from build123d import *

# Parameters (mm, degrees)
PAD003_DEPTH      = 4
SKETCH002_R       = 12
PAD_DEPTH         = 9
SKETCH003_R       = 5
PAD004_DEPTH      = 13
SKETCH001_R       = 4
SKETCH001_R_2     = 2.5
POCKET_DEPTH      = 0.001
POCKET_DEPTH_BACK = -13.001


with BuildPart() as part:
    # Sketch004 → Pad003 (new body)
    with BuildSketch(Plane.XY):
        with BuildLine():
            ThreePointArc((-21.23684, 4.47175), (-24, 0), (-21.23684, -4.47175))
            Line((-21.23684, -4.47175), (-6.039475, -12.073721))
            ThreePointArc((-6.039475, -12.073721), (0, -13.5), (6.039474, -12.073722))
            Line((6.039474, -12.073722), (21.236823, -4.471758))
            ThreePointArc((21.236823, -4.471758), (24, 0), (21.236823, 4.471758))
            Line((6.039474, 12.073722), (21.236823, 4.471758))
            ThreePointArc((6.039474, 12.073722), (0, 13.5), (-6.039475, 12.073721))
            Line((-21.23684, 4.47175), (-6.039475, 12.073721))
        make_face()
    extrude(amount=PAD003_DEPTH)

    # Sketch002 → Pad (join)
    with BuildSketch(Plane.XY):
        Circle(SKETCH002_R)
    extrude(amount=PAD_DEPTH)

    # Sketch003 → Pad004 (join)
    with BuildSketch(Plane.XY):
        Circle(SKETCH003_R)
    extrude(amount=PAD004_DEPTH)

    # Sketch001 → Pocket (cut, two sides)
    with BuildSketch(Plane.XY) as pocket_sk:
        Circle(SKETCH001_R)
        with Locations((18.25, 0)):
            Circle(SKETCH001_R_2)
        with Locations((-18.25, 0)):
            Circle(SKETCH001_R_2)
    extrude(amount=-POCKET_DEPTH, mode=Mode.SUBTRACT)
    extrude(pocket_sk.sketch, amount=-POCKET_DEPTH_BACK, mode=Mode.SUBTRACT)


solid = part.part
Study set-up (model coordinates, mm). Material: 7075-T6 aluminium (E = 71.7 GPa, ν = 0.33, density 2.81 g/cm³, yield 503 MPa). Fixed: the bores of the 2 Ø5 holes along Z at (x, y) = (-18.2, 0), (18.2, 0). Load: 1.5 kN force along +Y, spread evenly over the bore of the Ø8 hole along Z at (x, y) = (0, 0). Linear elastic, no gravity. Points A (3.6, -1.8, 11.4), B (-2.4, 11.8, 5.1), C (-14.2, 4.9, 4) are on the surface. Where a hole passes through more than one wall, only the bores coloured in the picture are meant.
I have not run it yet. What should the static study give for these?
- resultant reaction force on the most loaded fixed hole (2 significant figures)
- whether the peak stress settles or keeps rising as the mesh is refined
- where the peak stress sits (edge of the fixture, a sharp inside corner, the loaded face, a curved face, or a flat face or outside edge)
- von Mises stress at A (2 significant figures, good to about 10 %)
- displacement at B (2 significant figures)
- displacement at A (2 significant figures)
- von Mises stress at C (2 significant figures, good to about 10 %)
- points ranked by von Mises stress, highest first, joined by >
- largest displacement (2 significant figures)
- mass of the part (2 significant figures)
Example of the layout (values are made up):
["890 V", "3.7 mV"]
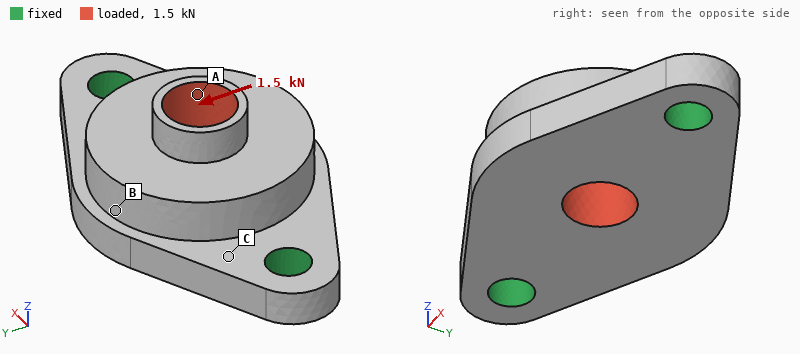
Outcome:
["750 N", "keeps rising", "edge of the fixture", "31 MPa", "31 µm", "31 µm", "58 MPa", "C > A > B", "40 µm", "15 g"]
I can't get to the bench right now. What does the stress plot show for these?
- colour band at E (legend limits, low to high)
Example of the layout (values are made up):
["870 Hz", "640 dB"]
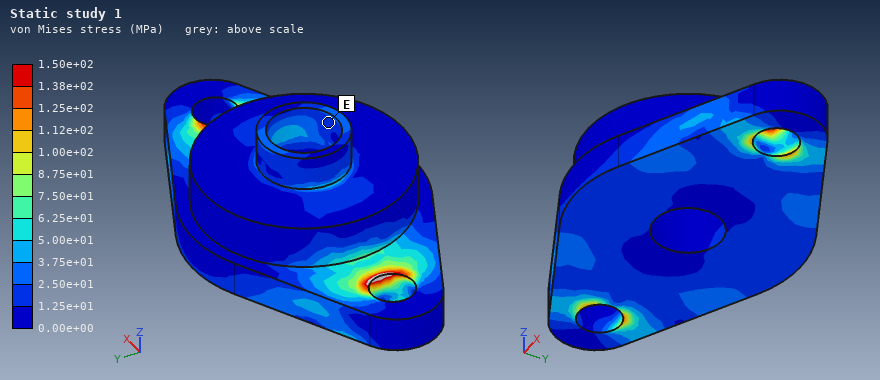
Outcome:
["1.25e+01 to 2.50e+01 MPa"]
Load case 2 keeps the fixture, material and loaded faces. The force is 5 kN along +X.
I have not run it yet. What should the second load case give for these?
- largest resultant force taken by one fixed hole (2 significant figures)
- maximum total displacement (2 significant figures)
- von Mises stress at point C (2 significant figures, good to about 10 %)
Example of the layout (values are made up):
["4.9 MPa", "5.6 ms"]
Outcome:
["2.6 kN", "30 µm", "41 MPa"]
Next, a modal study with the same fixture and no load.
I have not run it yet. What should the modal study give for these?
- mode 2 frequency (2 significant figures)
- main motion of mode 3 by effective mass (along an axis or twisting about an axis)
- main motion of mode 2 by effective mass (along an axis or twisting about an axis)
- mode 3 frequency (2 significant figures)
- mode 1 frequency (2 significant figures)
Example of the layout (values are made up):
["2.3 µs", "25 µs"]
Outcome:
["15 kHz", "along Y", "along Z", "26 kHz", "10000 Hz"]
